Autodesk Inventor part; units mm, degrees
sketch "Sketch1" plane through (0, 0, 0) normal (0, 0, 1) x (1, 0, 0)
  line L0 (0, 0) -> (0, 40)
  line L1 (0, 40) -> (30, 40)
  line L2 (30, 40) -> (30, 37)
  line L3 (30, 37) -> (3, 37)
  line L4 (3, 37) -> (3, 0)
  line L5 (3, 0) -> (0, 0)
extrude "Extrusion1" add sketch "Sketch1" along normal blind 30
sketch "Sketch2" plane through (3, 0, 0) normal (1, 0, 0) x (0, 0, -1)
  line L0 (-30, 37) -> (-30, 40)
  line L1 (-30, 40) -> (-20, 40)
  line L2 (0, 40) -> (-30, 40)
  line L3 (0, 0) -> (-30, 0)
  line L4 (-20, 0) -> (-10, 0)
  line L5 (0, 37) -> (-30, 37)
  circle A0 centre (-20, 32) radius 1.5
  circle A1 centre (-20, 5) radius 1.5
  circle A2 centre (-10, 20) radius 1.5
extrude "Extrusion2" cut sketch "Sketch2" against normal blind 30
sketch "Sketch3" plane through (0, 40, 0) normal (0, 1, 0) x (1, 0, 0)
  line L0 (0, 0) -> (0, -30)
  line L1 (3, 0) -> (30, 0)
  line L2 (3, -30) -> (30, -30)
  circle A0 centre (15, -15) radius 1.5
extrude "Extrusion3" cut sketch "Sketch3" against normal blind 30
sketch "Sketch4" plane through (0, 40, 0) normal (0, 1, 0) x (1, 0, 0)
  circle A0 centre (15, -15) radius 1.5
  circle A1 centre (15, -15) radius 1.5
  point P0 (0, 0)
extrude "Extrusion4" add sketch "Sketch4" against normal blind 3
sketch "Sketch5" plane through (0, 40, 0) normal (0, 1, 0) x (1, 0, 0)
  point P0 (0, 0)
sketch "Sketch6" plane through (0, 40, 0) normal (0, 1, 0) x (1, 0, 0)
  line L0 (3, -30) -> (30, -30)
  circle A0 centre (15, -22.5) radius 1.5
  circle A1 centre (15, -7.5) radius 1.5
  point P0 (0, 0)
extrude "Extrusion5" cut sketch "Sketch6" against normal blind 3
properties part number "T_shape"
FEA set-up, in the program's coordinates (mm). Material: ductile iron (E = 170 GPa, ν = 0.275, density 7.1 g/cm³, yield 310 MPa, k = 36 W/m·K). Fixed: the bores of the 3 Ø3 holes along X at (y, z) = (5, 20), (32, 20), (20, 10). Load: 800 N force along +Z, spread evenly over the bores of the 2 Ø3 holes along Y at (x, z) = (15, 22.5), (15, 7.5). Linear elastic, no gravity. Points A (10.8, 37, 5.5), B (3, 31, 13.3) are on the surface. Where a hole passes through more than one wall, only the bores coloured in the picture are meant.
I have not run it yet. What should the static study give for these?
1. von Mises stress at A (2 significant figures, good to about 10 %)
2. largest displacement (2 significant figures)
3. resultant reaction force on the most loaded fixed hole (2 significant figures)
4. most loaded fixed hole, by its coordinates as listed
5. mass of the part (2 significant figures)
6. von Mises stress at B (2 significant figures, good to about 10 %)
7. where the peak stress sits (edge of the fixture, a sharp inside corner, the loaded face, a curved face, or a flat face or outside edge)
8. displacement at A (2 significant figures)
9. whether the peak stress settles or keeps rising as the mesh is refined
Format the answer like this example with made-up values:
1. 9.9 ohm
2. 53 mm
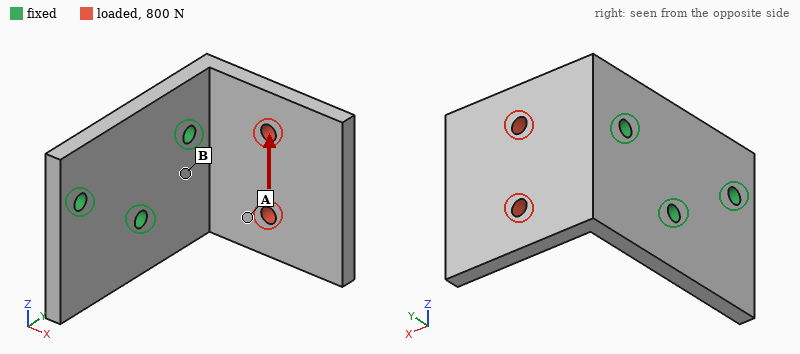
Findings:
1. 38 MPa
2. 0.15 mm
3. 890 N
4. (32, 20)
5. 42 g
6. 110 MPa
7. edge of the fixture
8. 0.068 mm
9. keeps rising
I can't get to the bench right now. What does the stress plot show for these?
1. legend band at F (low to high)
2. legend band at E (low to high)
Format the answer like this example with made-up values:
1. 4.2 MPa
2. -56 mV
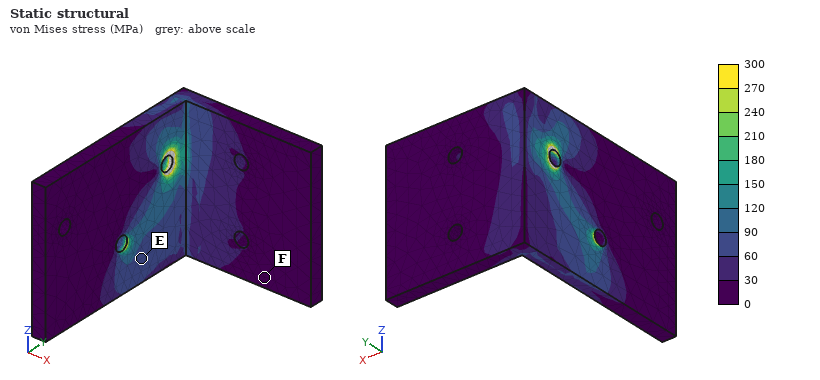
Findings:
1. 0 to 30 MPa
2. 60 to 90 MPa
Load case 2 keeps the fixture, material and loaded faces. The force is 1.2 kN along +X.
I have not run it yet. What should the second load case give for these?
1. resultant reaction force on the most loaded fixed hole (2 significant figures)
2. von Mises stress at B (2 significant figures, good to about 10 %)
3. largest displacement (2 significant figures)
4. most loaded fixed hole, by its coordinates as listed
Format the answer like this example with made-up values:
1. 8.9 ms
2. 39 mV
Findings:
1. 1.2 kN
2. 110 MPa
3. 0.15 mm
4. (32, 20)
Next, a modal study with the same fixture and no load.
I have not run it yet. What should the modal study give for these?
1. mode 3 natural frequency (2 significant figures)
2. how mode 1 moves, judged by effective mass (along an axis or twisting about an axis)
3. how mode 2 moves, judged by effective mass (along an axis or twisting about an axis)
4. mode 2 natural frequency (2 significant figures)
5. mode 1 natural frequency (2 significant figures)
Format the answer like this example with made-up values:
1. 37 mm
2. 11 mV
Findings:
1. 6200 Hz
2. along Y
3. along Z
4. 3300 Hz
5. 2000 Hz
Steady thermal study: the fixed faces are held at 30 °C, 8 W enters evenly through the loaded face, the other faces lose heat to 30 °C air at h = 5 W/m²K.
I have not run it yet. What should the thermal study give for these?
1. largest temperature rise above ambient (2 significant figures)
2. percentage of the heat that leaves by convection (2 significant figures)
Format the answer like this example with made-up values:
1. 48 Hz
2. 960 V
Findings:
1. 60 K
2. 6.5 %
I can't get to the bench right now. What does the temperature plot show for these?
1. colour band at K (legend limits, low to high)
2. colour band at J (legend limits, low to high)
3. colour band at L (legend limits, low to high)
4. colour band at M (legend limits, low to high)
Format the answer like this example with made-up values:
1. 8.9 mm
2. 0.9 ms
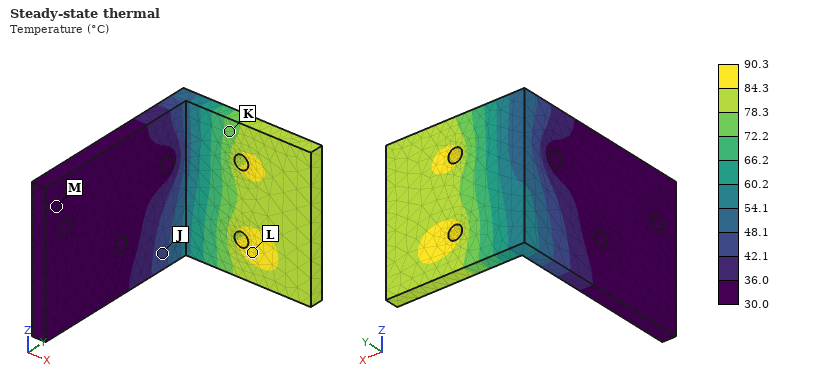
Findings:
1. 72.2 to 78.3 °C
2. 42.1 to 48.1 °C
3. 84.3 to 90.3 °C
4. 30.0 to 36.0 °C
